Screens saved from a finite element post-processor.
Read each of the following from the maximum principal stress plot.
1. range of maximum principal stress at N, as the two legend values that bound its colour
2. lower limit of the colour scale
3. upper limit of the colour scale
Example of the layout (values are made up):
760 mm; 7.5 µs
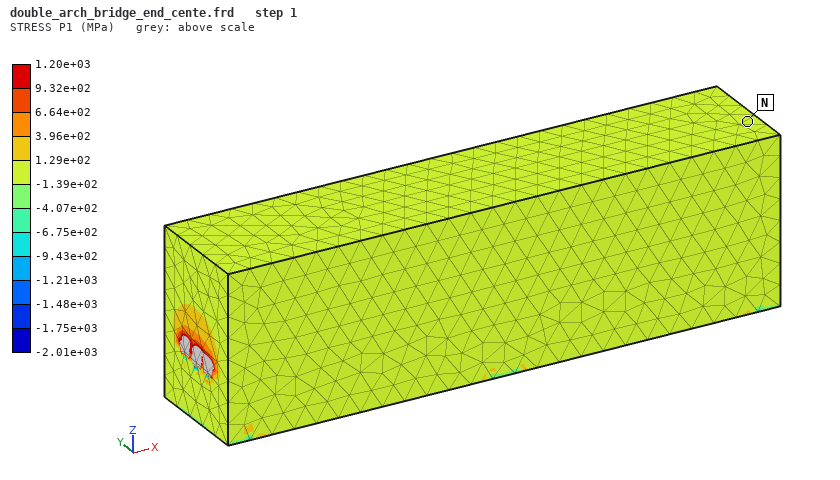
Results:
-1.39e+02 to 1.29e+02 MPa; -2.01e+03 MPa; 1.20e+03 MPa
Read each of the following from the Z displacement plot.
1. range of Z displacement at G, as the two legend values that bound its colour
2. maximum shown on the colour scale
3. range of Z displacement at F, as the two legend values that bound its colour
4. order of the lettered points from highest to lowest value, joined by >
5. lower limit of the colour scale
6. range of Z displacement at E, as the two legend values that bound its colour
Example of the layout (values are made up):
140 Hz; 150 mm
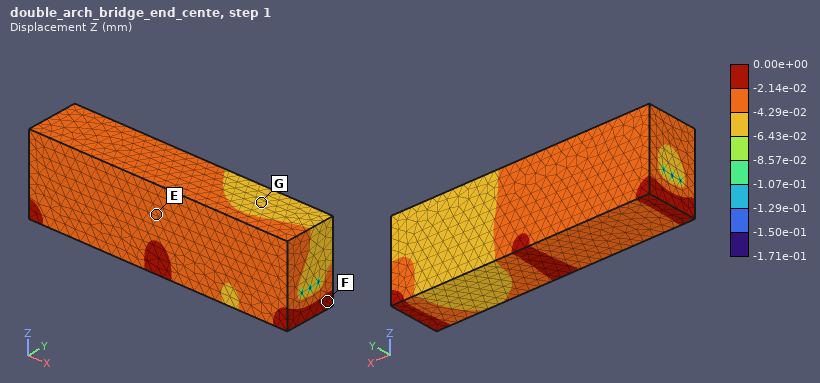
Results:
-6.43e-02 to -4.29e-02 mm; 0.00e+00 mm; -2.14e-02 to 0.00e+00 mm; F > E > G; -1.71e-01 mm; -4.29e-02 to -2.14e-02 mm
